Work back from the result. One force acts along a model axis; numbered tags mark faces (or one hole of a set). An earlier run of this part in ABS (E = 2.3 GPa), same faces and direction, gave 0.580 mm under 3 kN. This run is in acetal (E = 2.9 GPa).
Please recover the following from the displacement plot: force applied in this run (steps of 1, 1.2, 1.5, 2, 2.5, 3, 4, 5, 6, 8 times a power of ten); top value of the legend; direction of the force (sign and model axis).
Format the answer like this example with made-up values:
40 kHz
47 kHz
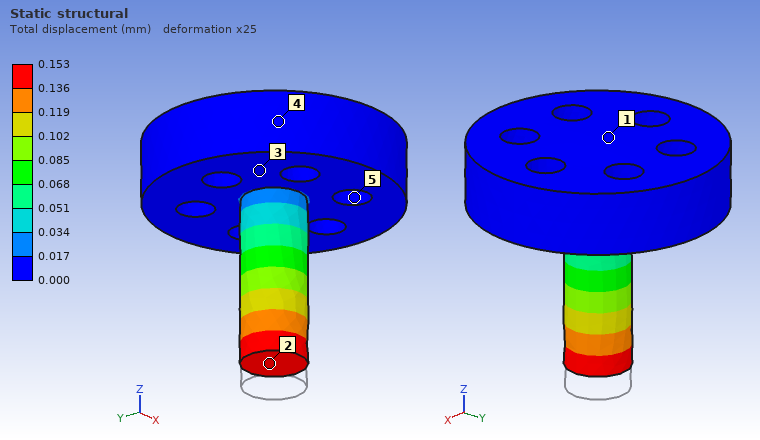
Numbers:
1 kN
0.153 mm
+Z
